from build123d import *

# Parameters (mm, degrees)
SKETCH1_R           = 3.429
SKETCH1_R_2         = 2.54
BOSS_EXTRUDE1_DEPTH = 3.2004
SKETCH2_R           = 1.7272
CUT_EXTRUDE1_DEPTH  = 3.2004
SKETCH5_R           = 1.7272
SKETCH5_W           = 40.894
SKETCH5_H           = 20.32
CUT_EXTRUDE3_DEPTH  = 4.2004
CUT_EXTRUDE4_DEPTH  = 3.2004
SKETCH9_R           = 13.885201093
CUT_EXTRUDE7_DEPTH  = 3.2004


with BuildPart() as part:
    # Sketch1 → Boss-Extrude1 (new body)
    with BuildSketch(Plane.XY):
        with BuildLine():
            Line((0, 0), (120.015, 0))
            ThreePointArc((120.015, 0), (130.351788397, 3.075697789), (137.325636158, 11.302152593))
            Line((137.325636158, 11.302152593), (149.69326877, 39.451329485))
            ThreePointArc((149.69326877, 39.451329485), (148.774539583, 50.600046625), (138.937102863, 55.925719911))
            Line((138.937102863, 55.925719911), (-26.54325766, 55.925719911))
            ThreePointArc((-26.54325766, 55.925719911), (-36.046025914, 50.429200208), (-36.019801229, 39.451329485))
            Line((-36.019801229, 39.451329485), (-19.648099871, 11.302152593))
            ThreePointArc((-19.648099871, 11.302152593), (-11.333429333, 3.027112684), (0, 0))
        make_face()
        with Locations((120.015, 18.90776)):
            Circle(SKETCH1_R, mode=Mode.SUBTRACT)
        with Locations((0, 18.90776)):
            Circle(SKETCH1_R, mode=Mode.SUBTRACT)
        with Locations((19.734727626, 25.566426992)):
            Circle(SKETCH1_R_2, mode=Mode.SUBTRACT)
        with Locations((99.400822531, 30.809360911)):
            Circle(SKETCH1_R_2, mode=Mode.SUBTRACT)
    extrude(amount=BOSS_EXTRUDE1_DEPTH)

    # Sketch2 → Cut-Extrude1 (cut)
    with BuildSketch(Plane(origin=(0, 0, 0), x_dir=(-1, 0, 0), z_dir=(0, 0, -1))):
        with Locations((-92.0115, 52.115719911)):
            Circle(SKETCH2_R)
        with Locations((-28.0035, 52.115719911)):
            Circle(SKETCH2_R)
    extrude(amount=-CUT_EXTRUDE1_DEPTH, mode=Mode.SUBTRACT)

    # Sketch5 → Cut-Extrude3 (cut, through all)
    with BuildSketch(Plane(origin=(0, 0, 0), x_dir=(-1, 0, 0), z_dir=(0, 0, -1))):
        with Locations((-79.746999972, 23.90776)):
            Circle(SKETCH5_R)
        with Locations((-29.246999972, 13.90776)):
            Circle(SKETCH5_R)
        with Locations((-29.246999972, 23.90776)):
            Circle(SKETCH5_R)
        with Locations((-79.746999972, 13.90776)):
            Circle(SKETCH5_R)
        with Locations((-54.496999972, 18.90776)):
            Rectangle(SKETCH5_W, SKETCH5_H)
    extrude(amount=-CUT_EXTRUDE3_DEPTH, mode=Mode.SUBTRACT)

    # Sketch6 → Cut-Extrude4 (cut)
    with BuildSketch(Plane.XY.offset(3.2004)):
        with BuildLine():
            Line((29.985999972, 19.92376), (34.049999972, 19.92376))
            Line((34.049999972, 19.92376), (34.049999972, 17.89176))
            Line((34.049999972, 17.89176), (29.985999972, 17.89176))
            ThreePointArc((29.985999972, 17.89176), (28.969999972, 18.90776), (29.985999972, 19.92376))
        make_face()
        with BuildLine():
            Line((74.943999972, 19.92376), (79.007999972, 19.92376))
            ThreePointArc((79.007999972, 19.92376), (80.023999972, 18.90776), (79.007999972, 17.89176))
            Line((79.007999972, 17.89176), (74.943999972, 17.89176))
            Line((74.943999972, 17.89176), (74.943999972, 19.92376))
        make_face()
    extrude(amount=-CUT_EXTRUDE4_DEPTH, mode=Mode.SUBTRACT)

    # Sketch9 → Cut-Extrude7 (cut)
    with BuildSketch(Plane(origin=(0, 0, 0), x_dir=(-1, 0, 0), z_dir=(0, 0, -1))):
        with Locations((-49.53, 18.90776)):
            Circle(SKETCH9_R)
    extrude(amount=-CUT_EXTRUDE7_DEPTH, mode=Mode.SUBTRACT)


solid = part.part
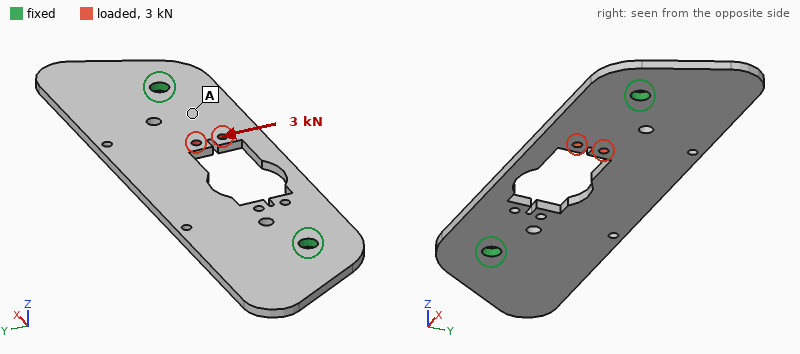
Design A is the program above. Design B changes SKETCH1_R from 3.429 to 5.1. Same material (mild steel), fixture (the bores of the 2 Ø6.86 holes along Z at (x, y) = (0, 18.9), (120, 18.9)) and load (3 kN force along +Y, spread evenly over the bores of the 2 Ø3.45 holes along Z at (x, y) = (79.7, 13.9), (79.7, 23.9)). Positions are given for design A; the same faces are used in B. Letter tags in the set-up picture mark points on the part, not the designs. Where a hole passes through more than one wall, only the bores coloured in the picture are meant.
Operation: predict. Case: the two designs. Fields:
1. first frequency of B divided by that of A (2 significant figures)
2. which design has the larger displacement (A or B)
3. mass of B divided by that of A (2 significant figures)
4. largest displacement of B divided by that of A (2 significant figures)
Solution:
1.1
A
0.99
0.89
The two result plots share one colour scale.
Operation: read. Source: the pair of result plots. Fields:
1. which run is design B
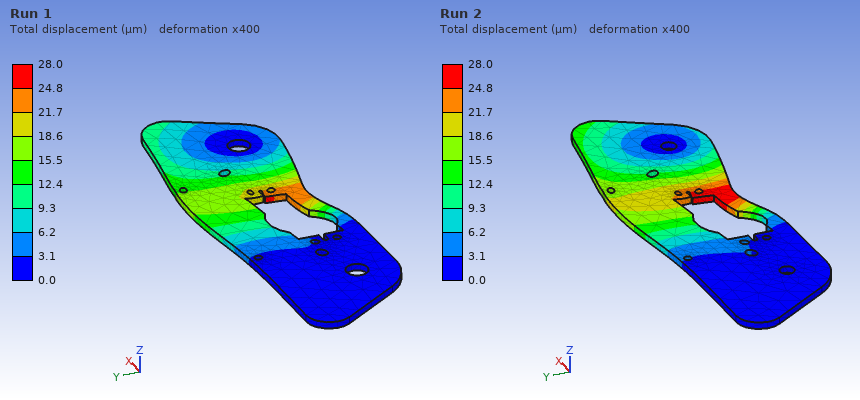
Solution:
Run 1
